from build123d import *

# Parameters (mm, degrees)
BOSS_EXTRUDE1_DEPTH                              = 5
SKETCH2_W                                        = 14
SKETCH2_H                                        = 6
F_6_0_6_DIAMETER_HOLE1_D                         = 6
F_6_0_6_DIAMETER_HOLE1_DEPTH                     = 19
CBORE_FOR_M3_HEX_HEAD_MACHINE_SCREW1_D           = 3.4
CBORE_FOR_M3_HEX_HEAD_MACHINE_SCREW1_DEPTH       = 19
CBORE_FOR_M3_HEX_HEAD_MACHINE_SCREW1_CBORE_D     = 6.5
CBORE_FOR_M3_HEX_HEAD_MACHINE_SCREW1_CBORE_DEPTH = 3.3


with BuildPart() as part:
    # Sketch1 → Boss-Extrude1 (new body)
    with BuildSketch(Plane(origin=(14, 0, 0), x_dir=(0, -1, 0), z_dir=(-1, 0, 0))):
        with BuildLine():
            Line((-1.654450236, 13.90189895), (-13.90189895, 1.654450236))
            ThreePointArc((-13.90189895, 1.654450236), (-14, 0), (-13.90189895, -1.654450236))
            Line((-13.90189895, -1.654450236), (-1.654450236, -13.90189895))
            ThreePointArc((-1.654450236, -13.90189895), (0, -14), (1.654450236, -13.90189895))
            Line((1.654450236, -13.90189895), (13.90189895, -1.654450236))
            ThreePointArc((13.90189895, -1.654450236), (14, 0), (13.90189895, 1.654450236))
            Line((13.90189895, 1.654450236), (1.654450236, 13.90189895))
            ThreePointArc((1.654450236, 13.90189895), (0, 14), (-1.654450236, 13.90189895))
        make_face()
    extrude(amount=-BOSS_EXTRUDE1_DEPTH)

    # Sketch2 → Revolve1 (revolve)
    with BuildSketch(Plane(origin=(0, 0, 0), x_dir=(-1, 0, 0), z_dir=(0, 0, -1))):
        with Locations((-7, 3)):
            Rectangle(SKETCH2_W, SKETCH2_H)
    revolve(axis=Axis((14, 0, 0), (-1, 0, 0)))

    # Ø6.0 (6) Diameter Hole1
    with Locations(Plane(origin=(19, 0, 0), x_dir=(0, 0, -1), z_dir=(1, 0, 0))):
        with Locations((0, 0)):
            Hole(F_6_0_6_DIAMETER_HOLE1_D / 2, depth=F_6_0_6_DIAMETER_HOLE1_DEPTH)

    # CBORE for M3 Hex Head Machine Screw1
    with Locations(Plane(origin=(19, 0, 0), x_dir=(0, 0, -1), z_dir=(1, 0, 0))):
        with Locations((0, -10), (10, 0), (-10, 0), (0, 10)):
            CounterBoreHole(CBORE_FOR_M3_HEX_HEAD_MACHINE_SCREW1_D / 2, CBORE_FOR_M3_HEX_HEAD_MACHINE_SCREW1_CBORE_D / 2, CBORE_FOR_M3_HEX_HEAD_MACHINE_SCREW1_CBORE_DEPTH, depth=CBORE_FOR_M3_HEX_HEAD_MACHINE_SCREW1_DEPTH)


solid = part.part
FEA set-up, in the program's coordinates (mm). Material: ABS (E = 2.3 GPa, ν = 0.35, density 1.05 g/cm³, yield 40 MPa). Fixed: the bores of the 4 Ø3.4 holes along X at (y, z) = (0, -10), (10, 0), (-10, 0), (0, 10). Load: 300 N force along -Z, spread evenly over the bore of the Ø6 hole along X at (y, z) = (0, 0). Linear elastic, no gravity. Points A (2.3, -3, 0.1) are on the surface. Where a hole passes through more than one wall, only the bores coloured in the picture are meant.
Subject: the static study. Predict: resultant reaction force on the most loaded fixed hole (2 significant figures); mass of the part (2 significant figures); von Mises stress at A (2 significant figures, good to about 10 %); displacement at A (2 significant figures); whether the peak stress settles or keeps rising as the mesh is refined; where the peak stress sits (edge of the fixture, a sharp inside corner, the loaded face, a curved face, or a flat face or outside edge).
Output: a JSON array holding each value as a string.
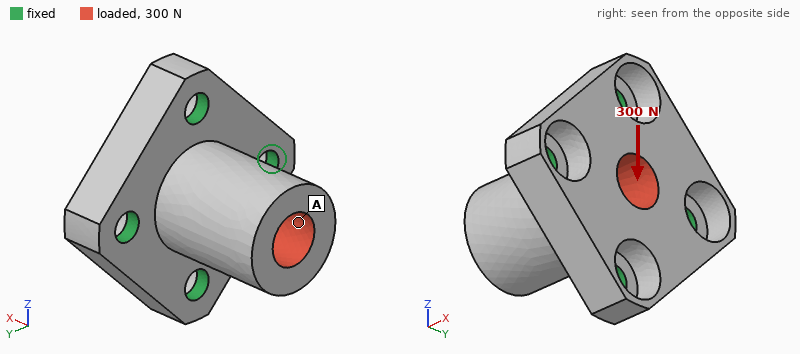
["120 N", "3.1 g", "2.8 MPa", "0.14 mm", "keeps rising", "edge of the fixture"]
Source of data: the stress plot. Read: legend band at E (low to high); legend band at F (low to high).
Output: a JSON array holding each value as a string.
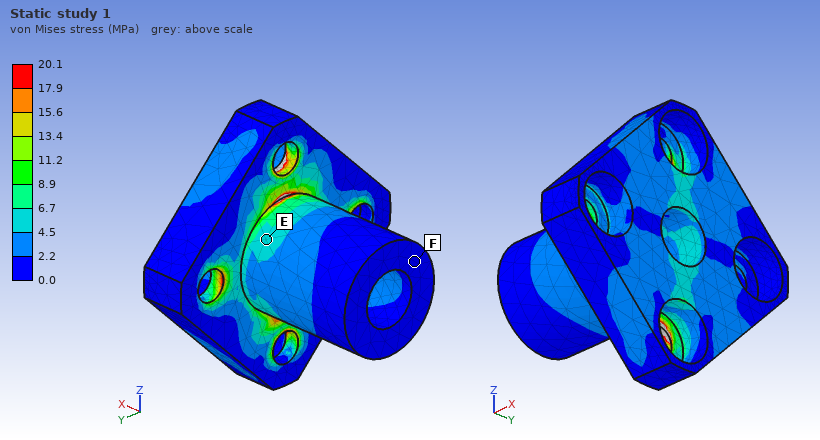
["4.5 to 6.7 MPa", "0.0 to 2.2 MPa"]
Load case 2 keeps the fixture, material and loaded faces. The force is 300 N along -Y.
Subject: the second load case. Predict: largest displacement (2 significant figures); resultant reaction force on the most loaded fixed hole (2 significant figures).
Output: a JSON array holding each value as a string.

["0.17 mm", "120 N"]
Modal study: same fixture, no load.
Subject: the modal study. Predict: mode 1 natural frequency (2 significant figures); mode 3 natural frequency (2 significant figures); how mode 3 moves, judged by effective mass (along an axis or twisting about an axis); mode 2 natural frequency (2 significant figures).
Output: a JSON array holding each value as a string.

["6100 Hz", "10 kHz", "along X", "6100 Hz"]
